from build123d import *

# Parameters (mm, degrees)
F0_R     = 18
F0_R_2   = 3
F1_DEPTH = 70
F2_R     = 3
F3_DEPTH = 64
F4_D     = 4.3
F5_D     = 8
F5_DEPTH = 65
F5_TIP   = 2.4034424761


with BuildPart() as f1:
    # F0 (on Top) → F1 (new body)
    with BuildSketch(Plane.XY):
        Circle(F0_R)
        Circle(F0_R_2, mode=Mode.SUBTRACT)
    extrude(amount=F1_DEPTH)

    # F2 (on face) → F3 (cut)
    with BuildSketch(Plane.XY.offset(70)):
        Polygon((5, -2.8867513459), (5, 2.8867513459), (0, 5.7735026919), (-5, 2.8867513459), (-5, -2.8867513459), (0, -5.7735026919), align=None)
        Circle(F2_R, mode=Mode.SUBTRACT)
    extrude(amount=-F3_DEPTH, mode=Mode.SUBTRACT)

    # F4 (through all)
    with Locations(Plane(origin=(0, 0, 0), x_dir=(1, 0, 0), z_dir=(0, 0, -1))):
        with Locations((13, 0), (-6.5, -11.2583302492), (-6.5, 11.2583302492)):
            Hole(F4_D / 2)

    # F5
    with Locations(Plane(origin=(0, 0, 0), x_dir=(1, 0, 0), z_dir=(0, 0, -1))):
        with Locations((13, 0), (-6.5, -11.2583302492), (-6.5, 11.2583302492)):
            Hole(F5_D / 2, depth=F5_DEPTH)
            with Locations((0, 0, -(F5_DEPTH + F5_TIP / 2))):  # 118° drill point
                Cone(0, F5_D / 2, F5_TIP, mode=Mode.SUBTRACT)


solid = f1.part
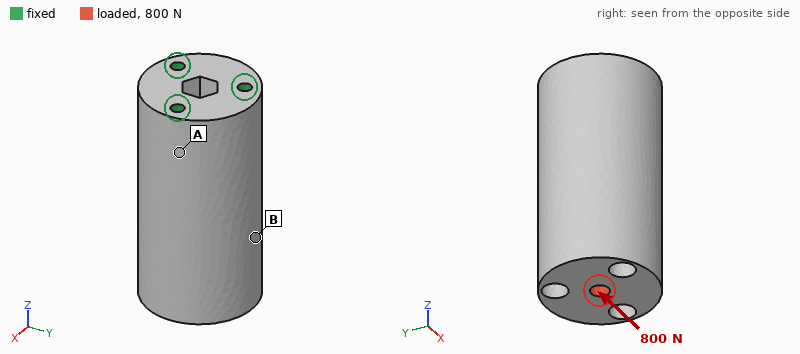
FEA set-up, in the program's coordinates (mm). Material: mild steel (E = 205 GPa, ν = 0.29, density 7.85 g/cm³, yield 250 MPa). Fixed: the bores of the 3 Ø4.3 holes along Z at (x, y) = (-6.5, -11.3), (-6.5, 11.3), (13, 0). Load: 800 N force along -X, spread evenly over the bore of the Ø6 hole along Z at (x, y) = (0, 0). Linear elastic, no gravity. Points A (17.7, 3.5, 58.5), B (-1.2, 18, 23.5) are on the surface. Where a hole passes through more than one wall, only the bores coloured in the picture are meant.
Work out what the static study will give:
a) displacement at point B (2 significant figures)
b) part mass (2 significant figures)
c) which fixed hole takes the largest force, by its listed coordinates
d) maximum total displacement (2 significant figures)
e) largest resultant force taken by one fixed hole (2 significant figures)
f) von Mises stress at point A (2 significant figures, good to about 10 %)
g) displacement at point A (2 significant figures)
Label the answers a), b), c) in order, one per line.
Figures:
a) 10.0 µm
b) 440 g
c) (13, 0)
d) 17 µm
e) 2.4 kN
f) 26 MPa
g) 3.3 µm
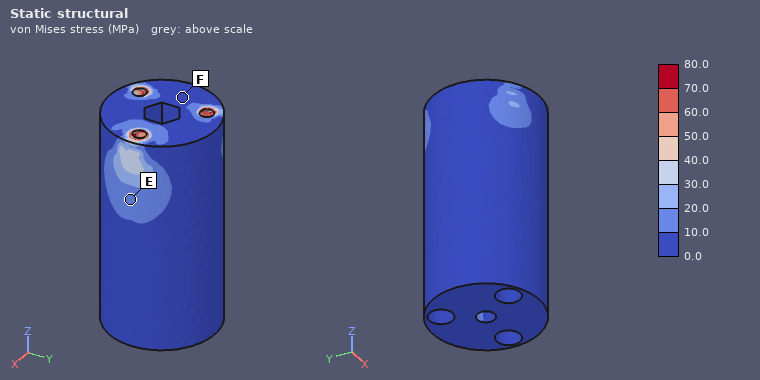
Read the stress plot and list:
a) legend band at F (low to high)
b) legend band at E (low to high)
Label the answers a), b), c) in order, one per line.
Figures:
a) 0.0 to 10.0 MPa
b) 10.0 to 20.0 MPa
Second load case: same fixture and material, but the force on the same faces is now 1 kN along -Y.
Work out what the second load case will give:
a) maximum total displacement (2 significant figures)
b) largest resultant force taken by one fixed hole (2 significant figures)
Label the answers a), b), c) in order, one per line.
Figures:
a) 22 µm
b) 2.6 kN
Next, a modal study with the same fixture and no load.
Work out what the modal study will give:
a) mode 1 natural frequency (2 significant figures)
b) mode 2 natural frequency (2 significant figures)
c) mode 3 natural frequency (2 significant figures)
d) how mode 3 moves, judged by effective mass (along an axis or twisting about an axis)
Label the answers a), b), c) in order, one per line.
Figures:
a) 2900 Hz
b) 2900 Hz
c) 9800 Hz
d) twisting about Z
